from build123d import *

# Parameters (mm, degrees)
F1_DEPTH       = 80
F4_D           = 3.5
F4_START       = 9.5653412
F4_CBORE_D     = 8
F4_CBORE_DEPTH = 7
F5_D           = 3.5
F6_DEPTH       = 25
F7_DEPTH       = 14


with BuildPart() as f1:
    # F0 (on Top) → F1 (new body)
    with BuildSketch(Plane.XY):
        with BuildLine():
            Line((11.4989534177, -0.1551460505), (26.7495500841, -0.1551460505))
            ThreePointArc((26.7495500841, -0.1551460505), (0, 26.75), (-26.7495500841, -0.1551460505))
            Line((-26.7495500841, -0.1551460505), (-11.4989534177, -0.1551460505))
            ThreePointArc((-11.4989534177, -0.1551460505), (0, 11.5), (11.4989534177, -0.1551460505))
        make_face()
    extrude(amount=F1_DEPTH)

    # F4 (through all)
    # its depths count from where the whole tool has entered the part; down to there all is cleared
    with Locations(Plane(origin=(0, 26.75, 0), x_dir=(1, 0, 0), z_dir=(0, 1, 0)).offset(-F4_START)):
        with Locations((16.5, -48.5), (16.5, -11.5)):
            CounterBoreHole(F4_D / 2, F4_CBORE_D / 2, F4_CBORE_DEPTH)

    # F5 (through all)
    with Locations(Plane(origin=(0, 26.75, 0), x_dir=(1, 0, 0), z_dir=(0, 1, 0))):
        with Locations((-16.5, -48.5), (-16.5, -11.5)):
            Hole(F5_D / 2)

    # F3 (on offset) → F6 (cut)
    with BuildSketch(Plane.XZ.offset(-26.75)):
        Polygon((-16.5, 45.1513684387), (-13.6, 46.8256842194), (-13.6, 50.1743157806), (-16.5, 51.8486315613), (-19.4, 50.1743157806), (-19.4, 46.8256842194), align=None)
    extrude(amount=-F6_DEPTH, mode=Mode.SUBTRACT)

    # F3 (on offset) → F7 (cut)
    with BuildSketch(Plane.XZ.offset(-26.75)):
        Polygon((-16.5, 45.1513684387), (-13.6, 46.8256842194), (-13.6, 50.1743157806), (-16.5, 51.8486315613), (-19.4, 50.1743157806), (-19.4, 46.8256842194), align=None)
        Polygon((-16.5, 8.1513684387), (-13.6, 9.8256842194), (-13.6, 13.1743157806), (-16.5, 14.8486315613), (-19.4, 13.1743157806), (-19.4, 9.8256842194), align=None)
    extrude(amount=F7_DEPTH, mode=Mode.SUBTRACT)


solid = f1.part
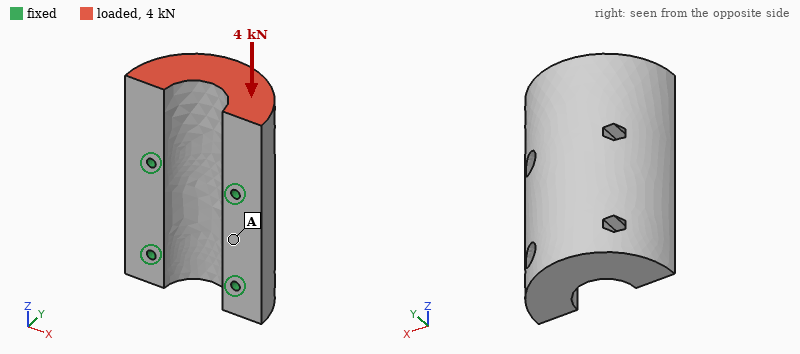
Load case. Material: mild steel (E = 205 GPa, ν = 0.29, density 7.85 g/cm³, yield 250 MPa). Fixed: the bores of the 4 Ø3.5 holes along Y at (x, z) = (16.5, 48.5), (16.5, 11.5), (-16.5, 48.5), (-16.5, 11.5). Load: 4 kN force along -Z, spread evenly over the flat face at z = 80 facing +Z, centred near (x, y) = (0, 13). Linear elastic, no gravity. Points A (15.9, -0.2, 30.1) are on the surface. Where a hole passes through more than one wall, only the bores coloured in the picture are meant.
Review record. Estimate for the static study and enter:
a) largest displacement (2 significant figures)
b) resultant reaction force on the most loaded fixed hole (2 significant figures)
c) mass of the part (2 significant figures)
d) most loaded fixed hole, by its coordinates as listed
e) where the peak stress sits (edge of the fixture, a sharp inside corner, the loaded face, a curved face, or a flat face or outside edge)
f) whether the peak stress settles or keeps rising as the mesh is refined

2.2 µm
1.6 kN
560 g
(-16.5, 48.5)
edge of the fixture
keeps rising
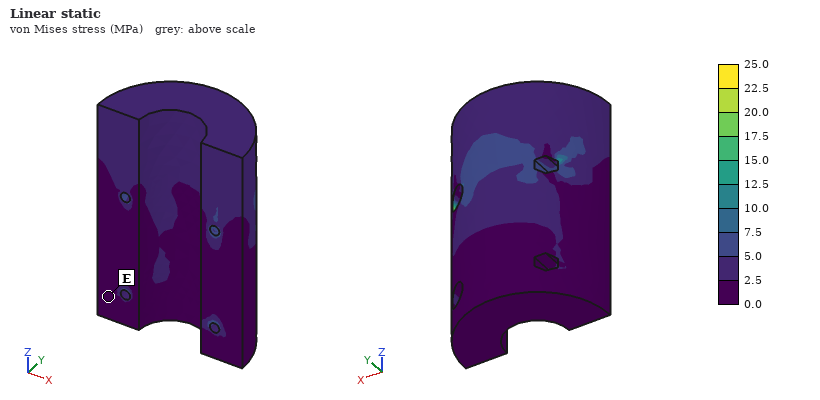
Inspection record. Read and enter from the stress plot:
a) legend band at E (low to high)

0.0 to 2.5 MPa
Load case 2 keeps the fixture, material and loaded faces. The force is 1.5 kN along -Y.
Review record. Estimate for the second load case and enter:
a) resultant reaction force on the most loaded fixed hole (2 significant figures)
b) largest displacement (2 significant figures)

1.4 kN
5.7 µm
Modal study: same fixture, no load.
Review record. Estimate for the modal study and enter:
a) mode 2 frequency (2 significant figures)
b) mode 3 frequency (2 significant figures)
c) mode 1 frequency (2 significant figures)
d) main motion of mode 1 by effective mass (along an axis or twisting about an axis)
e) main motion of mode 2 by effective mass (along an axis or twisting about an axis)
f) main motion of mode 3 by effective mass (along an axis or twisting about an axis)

12 kHz
16 kHz
9400 Hz
along Y
along X
along X
